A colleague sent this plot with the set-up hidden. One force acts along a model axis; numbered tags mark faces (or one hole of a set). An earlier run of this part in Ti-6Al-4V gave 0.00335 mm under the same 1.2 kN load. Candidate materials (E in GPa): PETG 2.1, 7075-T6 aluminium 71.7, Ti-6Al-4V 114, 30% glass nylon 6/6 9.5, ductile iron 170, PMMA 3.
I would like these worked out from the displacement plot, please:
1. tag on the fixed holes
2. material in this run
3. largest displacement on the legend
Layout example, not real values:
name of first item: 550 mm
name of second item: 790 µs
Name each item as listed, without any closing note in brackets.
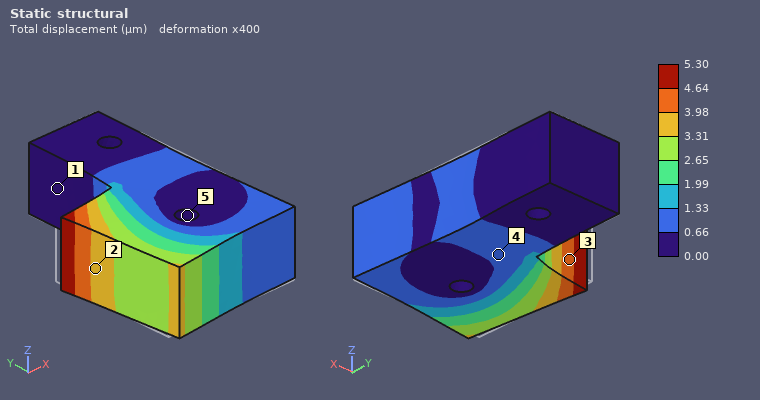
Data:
tag on the fixed holes: 5
material in this run: 7075-T6 aluminium
largest displacement on the legend: 5.30 µm
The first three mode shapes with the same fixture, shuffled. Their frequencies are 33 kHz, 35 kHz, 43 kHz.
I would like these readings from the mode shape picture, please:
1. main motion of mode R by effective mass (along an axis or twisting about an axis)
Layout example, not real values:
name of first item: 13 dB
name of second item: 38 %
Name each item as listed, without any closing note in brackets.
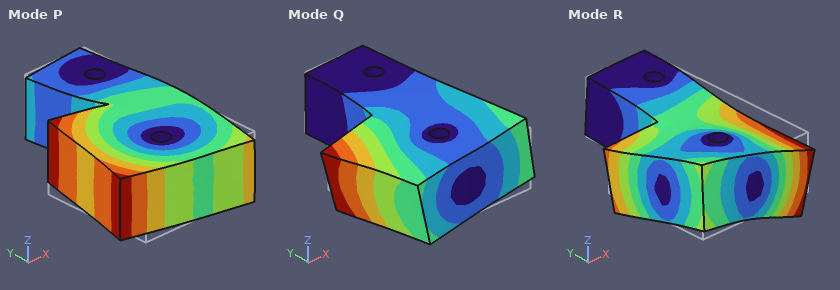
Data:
main motion of mode R by effective mass: along Z
